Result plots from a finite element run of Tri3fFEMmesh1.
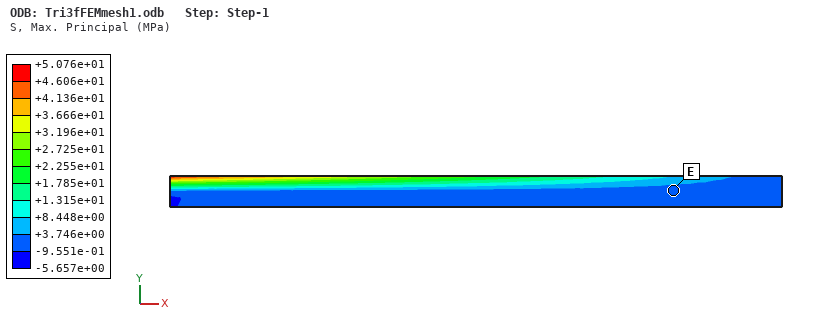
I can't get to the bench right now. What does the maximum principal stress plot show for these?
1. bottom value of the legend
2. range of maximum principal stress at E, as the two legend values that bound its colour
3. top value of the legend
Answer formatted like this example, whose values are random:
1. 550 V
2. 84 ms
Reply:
1. -5.657e+00 MPa
2. -9.551e-01 to +3.746e+00 MPa
3. +5.076e+01 MPa
